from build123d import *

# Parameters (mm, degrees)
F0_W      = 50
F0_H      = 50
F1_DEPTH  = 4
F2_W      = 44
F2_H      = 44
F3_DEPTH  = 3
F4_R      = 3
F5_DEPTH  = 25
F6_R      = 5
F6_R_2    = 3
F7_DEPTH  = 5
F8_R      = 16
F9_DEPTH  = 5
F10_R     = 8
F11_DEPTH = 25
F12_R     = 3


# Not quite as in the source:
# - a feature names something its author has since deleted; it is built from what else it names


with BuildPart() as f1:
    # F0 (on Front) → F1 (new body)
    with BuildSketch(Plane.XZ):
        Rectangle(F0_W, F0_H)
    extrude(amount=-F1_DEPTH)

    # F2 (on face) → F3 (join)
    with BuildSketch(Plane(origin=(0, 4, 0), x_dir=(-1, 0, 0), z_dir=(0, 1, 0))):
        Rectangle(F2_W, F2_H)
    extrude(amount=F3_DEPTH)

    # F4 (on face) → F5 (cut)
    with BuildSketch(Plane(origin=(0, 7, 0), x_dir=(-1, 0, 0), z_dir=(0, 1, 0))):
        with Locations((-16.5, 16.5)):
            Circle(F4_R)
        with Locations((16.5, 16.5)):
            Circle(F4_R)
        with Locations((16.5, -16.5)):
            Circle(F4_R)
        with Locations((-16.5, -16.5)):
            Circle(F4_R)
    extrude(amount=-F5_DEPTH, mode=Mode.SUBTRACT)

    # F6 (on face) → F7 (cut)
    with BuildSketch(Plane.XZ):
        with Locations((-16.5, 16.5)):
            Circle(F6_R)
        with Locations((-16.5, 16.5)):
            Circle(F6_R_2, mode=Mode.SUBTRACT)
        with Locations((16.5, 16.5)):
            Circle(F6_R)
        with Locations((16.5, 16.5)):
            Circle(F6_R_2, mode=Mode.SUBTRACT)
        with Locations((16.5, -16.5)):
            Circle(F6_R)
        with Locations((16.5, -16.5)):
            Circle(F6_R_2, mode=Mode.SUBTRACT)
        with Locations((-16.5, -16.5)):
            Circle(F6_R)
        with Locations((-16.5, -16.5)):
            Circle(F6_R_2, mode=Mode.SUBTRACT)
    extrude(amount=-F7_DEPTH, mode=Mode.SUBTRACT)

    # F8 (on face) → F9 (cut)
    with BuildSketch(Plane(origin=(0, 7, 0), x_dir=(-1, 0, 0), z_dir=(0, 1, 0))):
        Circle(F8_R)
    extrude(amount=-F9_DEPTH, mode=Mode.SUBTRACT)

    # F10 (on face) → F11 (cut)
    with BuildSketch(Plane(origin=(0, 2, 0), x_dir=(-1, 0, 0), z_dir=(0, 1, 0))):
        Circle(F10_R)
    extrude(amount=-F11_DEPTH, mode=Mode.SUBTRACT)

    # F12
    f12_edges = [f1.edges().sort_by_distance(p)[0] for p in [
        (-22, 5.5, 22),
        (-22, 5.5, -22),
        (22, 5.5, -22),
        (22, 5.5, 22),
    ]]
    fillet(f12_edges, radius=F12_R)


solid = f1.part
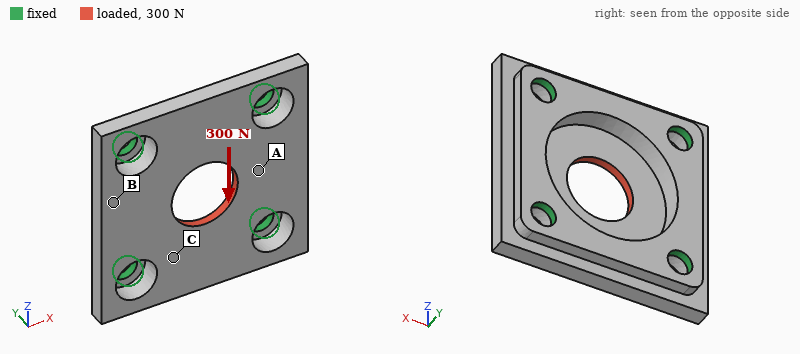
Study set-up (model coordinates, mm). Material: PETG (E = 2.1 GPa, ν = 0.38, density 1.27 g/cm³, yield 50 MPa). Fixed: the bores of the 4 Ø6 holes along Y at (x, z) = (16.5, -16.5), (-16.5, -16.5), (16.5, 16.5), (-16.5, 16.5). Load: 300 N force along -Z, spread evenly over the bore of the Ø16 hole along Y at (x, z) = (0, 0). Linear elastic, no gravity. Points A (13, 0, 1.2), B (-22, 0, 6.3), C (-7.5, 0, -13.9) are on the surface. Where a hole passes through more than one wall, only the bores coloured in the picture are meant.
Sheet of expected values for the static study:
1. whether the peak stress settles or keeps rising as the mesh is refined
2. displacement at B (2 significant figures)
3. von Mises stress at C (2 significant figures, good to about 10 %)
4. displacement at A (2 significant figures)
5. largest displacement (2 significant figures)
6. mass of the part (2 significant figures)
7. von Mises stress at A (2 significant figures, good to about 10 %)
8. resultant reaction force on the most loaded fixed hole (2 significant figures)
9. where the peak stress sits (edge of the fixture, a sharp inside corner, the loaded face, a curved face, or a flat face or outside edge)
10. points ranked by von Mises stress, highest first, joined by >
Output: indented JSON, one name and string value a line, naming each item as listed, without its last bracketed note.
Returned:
{
  "whether the peak stress settles or keeps rising as the mesh is refined": "keeps rising",
  "displacement at B": "9.1 µm",
  "von Mises stress at C": "3.3 MPa",
  "displacement at A": "19 µm",
  "largest displacement": "56 µm",
  "mass of the part": "12 g",
  "von Mises stress at A": "2.1 MPa",
  "resultant reaction force on the most loaded fixed hole": "77 N",
  "where the peak stress sits": "edge of the fixture",
  "points ranked by von Mises stress, highest first, joined by >": "C > A > B"
}
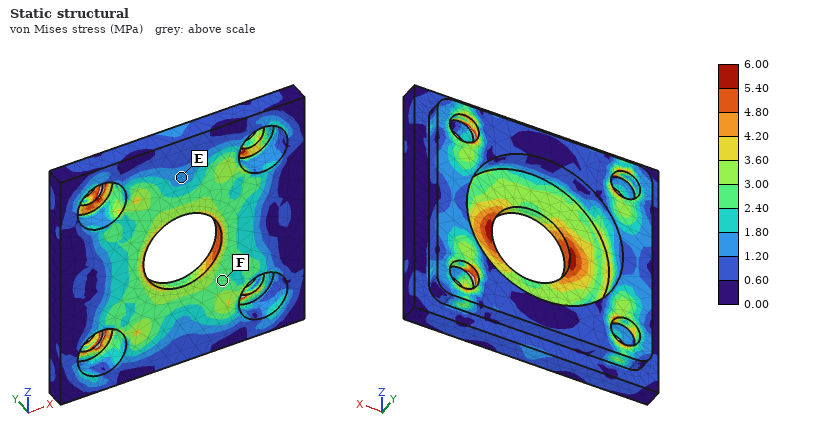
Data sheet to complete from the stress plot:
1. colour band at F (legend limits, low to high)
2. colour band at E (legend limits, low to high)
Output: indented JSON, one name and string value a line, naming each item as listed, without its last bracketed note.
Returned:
{
  "colour band at F": "2.40 to 3.00 MPa",
  "colour band at E": "1.20 to 1.80 MPa"
}
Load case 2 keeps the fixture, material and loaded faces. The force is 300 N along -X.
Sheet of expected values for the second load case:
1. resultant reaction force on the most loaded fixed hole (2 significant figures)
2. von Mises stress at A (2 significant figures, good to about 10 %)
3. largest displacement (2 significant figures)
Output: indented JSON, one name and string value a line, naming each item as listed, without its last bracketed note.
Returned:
{
  "resultant reaction force on the most loaded fixed hole": "77 N",
  "von Mises stress at A": "2.3 MPa",
  "largest displacement": "56 µm"
}
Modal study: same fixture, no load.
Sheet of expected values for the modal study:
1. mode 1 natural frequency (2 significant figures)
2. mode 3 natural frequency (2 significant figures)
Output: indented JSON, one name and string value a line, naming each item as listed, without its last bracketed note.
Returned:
{
  "mode 1 natural frequency": "5000 Hz",
  "mode 3 natural frequency": "5400 Hz"
}
